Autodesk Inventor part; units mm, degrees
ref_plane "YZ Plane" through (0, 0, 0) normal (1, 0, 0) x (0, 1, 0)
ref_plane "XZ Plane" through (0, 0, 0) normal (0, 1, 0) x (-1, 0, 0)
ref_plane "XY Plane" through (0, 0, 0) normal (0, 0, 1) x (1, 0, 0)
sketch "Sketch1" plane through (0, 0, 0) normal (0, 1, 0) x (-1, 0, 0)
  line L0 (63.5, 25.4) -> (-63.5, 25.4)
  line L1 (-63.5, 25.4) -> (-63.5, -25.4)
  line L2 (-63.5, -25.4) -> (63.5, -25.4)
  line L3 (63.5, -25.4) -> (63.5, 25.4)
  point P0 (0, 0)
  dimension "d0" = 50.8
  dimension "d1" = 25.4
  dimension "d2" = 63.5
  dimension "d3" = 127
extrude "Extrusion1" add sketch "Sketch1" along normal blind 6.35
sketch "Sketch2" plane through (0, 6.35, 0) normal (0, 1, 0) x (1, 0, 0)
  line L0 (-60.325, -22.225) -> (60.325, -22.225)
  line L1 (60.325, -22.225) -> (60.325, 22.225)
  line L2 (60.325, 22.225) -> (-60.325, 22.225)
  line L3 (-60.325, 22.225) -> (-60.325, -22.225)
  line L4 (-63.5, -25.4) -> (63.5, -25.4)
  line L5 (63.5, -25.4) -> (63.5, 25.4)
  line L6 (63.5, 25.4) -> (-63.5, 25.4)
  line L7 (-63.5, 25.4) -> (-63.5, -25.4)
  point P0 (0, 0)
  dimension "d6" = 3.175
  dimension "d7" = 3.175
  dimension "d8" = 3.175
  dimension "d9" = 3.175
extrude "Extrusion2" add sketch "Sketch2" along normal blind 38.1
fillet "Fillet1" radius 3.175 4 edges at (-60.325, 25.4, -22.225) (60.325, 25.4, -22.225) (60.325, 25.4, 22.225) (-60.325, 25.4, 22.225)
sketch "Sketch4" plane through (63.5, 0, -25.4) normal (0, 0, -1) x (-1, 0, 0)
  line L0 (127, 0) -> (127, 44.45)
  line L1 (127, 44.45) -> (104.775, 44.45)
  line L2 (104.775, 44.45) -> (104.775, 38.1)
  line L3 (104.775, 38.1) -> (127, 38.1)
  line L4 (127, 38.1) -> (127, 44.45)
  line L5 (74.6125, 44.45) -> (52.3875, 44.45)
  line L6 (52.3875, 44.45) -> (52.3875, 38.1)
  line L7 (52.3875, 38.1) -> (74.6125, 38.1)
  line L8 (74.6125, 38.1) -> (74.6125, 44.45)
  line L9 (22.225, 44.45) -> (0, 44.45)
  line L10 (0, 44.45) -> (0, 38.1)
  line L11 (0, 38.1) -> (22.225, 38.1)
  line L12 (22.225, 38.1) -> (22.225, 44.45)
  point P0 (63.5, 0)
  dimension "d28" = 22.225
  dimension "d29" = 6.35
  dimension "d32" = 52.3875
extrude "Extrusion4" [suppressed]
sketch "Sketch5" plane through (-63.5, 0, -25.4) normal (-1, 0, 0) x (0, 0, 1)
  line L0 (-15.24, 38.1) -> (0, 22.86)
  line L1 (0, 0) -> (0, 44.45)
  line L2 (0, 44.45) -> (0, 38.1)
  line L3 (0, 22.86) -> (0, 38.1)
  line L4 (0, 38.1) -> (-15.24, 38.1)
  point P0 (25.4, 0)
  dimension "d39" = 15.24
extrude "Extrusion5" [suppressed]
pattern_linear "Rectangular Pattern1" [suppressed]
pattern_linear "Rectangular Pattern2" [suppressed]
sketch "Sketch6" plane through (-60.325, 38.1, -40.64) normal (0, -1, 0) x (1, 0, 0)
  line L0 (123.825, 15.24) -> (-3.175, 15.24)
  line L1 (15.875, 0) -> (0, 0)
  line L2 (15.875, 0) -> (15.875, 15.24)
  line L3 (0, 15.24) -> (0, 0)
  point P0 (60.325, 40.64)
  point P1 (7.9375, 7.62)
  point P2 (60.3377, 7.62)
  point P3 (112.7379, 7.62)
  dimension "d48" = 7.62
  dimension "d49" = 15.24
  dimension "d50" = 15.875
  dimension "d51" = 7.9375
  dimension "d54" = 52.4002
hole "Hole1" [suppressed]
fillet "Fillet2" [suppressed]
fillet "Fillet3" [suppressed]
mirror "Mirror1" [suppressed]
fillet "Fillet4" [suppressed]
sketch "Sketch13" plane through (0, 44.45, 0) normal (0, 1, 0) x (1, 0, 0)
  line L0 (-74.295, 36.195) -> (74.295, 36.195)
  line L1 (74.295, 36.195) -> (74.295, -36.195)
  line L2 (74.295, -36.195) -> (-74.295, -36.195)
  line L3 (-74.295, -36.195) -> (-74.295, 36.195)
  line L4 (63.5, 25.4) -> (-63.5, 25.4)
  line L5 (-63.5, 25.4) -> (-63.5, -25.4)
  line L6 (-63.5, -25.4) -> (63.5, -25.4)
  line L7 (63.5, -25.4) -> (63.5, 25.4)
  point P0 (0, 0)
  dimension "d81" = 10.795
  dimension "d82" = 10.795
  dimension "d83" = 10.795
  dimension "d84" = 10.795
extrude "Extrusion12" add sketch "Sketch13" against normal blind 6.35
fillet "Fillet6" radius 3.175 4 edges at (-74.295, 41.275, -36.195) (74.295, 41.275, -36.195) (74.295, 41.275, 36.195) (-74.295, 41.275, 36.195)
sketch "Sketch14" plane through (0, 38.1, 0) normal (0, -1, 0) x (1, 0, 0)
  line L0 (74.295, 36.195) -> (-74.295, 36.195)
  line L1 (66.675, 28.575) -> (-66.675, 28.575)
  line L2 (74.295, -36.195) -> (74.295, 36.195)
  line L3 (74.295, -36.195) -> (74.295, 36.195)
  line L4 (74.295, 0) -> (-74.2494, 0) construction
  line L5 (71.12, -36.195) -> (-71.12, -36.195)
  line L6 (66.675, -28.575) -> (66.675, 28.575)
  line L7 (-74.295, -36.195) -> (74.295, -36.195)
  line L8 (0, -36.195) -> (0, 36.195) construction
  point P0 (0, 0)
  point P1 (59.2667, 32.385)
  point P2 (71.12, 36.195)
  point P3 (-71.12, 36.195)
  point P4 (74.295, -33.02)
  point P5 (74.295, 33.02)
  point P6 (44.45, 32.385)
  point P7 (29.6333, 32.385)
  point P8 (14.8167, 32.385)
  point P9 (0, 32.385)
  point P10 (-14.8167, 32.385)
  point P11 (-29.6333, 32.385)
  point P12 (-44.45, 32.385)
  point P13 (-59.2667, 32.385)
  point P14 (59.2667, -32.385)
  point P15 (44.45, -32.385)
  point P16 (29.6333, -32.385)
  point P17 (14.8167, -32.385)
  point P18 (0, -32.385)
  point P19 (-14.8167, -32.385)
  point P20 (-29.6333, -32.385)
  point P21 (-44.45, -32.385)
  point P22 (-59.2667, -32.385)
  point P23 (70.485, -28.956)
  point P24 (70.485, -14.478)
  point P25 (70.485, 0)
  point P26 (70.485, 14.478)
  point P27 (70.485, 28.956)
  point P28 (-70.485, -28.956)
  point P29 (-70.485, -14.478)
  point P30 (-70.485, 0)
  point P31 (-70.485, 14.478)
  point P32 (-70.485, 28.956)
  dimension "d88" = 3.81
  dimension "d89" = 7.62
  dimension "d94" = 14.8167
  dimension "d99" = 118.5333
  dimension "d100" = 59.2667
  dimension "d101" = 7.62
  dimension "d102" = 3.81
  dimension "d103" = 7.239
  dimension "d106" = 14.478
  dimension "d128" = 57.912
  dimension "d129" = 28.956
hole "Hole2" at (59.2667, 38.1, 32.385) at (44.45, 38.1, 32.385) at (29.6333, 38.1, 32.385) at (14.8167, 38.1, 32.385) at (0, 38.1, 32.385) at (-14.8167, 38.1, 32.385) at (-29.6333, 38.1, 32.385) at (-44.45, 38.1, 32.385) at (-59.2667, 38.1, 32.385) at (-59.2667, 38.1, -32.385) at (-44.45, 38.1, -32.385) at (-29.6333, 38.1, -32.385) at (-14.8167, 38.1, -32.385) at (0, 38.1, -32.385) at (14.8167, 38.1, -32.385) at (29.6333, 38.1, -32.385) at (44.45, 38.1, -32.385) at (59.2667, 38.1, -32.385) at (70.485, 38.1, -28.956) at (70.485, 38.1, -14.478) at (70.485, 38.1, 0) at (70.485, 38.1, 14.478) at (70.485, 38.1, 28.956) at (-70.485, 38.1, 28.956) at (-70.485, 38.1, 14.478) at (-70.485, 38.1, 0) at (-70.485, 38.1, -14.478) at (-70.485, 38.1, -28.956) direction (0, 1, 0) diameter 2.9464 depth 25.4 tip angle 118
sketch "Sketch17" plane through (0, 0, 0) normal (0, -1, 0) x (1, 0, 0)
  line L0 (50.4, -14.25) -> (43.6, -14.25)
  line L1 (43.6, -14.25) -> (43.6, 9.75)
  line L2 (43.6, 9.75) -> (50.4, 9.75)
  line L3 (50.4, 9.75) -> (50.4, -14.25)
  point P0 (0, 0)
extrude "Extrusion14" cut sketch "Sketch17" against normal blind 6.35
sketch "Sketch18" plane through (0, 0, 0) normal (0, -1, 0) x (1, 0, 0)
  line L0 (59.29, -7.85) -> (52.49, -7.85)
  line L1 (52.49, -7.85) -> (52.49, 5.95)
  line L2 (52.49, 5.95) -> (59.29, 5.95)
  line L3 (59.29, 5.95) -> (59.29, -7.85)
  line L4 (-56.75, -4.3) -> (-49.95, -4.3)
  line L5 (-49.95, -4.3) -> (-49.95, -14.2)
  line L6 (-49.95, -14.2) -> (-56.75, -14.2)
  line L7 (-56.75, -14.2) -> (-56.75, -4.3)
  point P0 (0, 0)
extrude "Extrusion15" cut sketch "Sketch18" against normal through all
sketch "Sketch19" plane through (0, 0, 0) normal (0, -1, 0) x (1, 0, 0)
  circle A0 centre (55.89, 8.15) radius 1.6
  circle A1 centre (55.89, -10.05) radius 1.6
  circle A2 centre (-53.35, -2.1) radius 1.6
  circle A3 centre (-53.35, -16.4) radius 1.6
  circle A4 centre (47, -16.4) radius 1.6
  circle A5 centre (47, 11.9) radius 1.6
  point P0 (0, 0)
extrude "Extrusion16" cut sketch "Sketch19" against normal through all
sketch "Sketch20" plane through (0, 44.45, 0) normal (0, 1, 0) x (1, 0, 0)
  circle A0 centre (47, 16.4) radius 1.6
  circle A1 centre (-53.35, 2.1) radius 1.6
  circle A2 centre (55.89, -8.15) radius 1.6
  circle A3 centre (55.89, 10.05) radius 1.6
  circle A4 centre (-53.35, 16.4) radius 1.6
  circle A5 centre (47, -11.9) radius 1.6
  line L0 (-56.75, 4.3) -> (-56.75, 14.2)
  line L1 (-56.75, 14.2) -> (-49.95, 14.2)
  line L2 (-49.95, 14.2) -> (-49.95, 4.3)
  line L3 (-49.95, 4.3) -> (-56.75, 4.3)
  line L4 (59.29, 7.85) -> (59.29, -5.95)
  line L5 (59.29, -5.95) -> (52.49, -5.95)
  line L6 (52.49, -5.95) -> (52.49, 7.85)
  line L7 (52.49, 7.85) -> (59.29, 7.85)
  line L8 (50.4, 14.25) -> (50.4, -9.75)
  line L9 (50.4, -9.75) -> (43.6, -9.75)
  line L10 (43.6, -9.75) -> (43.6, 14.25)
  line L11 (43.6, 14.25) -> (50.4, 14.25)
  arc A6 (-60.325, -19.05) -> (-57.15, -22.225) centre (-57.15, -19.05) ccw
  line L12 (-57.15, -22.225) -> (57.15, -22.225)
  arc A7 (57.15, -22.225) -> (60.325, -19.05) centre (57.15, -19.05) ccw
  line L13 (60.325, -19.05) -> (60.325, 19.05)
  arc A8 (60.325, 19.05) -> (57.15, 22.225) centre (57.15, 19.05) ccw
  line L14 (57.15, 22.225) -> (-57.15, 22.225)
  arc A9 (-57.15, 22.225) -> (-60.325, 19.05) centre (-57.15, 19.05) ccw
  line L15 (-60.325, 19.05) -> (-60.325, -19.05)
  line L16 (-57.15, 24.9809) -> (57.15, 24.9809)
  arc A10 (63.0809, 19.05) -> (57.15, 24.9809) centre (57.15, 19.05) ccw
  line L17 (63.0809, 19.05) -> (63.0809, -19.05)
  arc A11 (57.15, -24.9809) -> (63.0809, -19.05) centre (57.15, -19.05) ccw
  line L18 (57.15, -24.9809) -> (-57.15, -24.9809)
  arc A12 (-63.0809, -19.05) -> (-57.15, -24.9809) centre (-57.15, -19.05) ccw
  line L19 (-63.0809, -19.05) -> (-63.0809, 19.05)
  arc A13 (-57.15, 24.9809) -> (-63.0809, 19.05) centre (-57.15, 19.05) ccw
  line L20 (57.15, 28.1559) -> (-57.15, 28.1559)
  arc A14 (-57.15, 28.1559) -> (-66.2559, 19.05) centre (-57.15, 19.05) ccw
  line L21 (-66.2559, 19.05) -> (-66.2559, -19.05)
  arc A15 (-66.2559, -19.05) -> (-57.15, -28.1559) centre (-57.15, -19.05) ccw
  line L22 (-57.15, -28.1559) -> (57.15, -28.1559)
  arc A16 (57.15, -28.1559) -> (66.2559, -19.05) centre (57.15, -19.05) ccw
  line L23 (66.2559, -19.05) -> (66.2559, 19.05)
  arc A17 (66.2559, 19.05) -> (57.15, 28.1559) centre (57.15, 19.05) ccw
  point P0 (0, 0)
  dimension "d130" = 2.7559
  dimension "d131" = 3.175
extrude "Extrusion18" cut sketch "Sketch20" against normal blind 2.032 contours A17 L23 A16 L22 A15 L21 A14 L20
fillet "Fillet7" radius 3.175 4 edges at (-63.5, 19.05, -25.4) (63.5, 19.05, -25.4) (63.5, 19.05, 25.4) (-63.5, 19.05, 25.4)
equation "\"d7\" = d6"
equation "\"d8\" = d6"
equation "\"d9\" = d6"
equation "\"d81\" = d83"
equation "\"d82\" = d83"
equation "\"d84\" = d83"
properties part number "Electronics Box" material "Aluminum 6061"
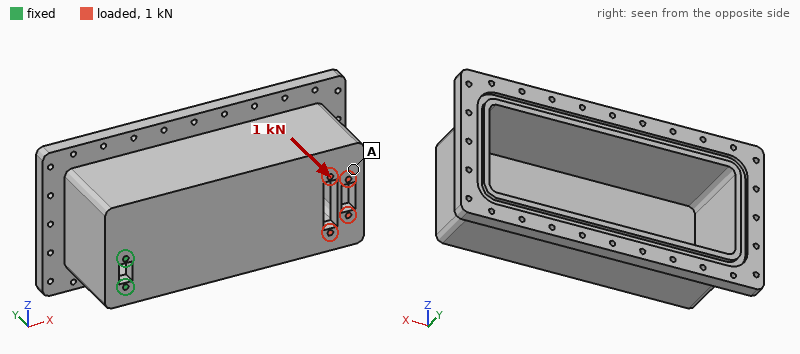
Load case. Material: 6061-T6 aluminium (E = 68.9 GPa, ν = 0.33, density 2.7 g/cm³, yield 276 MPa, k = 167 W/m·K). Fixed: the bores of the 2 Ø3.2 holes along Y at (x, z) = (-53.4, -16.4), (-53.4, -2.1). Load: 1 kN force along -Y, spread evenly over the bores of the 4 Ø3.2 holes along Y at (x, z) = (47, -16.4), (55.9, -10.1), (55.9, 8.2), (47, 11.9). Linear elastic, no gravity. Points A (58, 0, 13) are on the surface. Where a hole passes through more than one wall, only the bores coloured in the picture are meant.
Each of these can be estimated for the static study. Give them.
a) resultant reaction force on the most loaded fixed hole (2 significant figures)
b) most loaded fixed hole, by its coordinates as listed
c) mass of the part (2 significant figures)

740 N
(-53.4, -2.1)
280 g
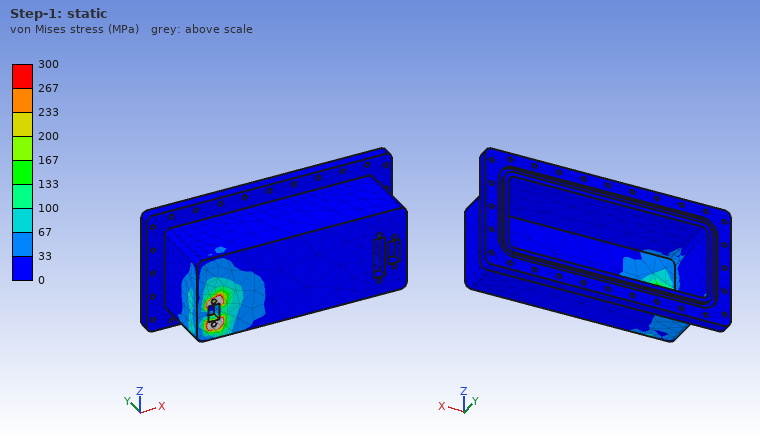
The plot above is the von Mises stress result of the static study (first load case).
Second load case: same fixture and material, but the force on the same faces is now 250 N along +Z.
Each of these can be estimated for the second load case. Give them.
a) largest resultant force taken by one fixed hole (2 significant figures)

1.4 kN
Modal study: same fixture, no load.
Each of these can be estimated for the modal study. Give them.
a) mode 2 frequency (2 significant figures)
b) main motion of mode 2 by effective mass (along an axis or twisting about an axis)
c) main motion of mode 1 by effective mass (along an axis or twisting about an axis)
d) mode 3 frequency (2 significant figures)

720 Hz
along Z
along Y
1300 Hz
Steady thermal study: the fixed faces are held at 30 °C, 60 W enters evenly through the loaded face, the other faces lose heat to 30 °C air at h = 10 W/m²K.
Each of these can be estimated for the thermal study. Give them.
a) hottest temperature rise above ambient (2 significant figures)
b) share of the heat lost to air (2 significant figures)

76 K
29 %
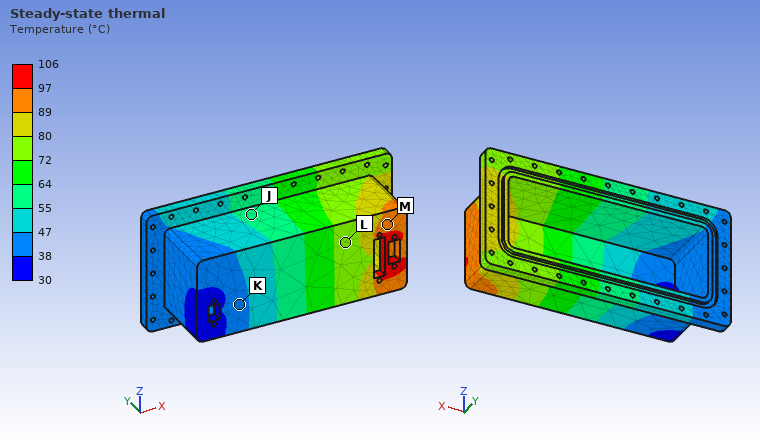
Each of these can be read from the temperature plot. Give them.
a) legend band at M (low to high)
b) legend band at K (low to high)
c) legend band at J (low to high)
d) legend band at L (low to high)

89 to 97 °C
38 to 47 °C
55 to 64 °C
72 to 80 °C
